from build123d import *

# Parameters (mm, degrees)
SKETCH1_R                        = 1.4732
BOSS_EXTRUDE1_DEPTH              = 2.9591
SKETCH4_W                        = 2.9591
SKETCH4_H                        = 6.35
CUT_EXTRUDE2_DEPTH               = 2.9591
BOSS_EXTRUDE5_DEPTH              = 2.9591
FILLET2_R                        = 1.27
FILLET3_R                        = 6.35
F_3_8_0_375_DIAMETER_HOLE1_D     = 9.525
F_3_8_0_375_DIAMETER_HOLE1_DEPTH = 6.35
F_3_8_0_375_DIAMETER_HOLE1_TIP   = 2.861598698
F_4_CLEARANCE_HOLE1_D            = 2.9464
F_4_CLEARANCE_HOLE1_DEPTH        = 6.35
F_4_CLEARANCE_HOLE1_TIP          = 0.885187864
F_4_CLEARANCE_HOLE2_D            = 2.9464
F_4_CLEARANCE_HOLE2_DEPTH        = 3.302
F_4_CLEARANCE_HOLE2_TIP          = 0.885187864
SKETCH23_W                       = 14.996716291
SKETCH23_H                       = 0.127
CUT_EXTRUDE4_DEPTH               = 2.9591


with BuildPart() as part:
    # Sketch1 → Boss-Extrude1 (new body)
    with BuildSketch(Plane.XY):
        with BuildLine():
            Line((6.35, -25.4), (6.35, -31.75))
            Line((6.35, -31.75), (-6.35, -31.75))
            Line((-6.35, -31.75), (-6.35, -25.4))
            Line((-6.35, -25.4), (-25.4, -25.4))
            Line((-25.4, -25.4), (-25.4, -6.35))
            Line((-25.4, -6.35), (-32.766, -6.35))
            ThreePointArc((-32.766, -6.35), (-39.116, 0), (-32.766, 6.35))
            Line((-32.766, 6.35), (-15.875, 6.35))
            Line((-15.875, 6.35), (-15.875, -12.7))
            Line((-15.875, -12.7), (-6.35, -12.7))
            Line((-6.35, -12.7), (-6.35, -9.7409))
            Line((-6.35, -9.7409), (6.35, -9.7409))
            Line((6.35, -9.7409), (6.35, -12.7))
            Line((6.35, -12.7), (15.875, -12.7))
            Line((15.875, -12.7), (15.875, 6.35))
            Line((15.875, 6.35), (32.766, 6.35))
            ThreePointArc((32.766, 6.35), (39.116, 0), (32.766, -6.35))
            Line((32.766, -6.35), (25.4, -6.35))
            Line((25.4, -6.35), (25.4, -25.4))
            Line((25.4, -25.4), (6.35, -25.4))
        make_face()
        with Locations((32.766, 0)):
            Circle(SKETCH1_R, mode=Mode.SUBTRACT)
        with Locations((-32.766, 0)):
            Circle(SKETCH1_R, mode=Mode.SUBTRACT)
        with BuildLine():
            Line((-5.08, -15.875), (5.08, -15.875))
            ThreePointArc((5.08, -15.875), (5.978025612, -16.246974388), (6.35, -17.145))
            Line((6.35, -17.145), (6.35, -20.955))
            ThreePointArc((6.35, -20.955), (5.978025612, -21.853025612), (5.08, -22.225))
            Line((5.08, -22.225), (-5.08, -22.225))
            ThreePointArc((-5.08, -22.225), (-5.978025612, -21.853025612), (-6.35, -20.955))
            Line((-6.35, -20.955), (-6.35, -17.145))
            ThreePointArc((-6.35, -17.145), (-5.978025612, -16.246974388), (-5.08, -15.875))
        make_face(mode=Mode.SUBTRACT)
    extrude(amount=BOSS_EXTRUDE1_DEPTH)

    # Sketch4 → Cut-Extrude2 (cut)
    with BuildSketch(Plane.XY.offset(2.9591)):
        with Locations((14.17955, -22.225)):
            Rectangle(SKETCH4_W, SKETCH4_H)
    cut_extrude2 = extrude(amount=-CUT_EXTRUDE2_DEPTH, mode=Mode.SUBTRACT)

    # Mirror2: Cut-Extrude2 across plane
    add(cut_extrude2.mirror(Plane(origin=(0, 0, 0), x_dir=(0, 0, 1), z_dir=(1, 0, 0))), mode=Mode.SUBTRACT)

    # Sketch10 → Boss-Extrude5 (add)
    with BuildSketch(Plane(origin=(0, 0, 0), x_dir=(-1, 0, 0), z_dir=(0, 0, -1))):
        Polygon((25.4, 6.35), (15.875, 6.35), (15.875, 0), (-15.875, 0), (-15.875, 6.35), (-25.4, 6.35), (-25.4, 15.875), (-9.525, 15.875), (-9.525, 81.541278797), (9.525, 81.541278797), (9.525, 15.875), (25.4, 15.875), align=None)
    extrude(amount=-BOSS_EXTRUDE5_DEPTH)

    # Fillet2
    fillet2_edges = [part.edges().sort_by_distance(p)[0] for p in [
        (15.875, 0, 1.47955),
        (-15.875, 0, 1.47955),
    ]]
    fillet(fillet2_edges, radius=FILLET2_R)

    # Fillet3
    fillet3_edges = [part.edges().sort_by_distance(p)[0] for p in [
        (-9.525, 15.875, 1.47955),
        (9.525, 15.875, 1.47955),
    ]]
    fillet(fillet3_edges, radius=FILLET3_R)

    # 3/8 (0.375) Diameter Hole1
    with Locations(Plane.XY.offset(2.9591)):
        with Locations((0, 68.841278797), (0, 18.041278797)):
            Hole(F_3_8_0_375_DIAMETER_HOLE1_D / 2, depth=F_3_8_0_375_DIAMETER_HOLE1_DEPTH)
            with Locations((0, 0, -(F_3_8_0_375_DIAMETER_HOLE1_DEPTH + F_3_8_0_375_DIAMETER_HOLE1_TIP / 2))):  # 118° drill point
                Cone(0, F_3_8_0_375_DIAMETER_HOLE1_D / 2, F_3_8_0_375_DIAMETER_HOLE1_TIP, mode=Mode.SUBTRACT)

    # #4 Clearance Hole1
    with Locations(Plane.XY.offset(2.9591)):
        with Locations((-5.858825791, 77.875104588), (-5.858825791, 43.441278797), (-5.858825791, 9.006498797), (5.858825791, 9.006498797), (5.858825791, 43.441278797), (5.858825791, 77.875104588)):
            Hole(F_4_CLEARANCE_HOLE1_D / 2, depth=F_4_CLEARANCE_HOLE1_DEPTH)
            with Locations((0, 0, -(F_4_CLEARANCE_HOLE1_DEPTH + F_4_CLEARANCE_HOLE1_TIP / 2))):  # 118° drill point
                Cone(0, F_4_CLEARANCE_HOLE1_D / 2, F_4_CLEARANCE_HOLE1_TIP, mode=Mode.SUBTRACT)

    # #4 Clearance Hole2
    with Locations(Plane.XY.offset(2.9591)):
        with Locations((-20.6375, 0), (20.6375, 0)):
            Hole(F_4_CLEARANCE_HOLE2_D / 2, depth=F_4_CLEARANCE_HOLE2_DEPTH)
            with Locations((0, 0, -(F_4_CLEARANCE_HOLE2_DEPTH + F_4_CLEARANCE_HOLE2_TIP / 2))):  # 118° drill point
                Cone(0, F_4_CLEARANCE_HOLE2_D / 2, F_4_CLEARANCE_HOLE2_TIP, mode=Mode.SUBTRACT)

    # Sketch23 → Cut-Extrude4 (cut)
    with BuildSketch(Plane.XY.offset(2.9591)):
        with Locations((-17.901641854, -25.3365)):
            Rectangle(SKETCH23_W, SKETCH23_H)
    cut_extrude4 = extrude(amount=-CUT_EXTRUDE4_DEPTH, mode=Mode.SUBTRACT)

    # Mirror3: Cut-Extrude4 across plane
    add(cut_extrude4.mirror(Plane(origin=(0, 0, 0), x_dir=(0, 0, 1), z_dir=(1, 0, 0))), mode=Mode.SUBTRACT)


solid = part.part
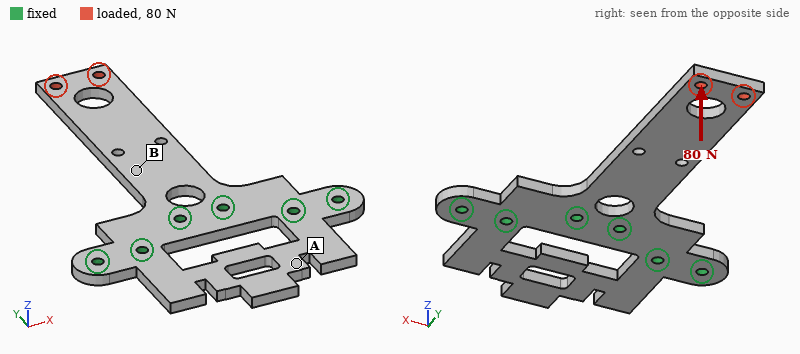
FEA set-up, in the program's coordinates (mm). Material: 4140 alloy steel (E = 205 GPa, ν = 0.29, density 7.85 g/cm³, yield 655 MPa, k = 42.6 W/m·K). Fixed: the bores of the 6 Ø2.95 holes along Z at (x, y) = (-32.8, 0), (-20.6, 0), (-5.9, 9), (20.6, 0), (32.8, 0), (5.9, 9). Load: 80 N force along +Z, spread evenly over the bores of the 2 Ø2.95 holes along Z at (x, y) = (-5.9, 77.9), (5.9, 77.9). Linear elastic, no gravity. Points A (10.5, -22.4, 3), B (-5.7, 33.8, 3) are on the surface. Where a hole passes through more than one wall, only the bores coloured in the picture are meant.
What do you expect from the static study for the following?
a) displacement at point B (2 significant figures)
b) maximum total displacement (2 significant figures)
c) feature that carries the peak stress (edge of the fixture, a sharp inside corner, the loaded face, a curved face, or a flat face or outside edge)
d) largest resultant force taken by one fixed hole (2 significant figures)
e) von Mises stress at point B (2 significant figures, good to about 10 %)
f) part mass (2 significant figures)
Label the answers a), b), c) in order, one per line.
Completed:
a) 0.19 mm
b) 1.3 mm
c) a curved face
d) 96 N
e) 130 MPa
f) 71 g
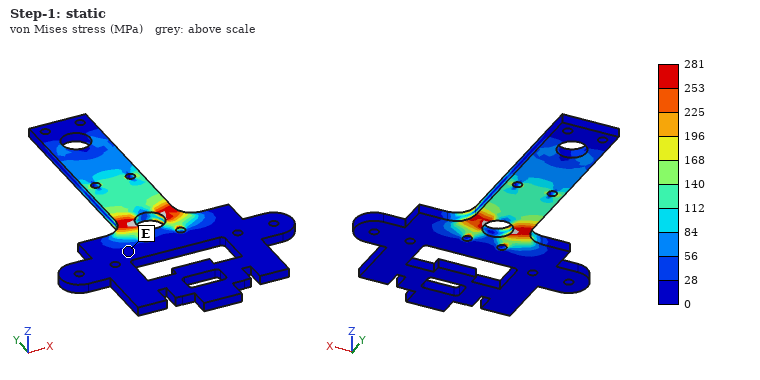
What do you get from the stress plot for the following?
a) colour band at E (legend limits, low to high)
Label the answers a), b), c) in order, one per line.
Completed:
a) 0 to 28 MPa
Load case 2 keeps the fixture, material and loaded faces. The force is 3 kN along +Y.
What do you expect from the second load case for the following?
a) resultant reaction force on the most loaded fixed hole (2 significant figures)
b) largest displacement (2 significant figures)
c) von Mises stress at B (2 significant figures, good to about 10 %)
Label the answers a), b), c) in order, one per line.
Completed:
a) 1.1 kN
b) 26 µm
c) 53 MPa
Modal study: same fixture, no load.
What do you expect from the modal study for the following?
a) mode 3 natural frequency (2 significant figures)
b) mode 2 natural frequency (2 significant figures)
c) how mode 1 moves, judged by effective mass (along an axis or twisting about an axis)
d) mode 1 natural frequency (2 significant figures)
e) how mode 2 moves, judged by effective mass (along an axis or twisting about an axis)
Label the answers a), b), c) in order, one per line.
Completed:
a) 2900 Hz
b) 2200 Hz
c) along Z
d) 480 Hz
e) along Z
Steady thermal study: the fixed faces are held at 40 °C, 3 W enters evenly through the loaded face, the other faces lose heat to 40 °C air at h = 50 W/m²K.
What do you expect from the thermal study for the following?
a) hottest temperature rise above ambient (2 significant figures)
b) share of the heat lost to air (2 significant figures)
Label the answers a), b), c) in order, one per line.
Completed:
a) 44 K
b) 82 %
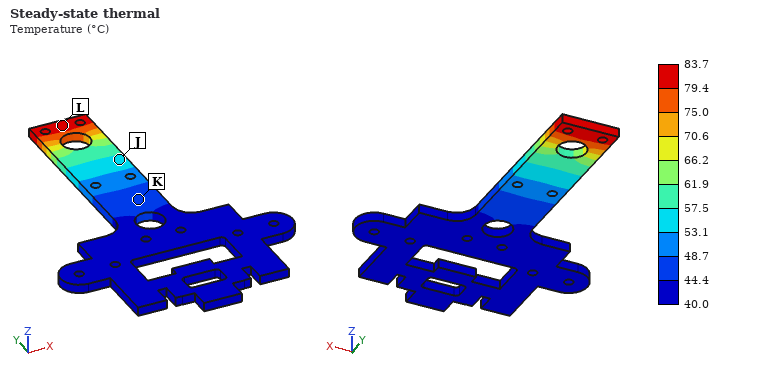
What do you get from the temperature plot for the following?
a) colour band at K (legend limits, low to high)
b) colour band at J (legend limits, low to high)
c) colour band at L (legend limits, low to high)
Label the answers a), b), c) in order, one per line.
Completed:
a) 44.4 to 48.7 °C
b) 53.1 to 57.5 °C
c) 79.4 to 83.7 °C
